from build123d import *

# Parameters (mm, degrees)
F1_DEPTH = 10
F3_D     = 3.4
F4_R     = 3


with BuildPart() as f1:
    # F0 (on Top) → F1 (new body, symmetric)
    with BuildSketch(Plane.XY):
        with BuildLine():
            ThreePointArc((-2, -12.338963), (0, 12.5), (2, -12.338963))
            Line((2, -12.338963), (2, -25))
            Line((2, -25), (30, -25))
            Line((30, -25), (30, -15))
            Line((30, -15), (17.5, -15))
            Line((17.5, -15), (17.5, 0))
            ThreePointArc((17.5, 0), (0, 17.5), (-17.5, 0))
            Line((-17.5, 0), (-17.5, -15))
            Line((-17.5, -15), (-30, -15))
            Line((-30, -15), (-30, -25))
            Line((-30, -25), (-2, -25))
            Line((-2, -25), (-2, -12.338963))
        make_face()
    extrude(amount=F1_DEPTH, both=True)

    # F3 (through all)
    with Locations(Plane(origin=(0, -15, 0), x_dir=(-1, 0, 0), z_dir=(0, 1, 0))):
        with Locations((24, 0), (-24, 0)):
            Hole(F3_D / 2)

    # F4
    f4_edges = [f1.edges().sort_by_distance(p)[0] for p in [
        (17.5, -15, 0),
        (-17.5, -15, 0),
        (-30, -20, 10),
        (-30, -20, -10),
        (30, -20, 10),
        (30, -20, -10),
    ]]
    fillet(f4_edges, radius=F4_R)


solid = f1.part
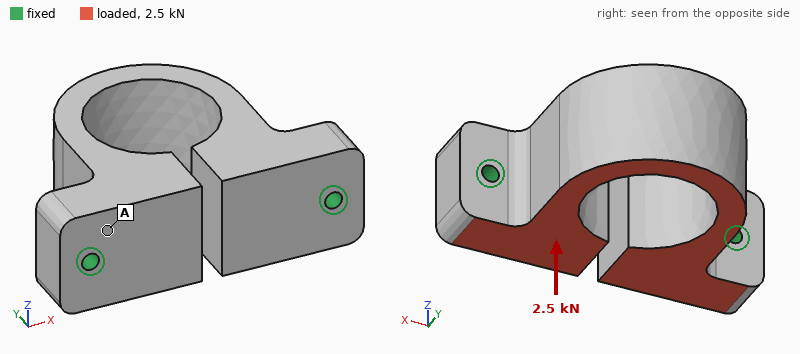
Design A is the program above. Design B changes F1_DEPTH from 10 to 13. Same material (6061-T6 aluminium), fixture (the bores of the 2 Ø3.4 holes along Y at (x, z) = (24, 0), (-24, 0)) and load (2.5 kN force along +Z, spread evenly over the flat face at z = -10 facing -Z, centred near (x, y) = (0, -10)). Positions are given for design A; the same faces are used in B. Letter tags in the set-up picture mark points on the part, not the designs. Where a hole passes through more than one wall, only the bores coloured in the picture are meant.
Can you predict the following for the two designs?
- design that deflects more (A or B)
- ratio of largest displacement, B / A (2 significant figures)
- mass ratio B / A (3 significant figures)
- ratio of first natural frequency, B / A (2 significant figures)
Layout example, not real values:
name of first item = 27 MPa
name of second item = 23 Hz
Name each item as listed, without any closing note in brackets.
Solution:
design that deflects more = A
ratio of largest displacement, B / A = 0.83
mass ratio B / A = 1.30
ratio of first natural frequency, B / A = 0.94
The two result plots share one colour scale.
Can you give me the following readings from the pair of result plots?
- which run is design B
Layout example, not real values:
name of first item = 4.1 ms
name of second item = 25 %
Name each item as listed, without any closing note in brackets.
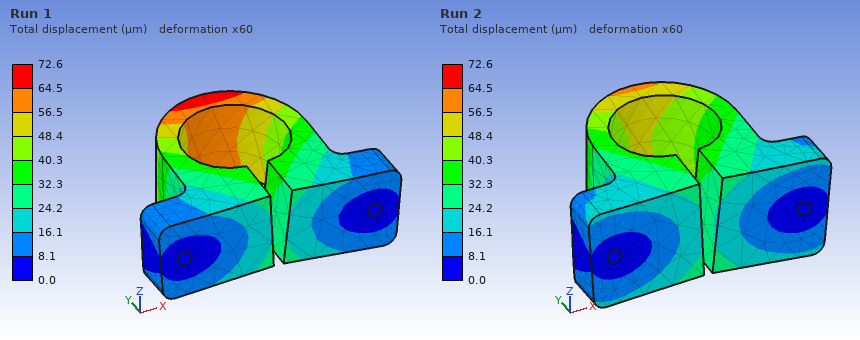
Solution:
which run is design B = Run 2
